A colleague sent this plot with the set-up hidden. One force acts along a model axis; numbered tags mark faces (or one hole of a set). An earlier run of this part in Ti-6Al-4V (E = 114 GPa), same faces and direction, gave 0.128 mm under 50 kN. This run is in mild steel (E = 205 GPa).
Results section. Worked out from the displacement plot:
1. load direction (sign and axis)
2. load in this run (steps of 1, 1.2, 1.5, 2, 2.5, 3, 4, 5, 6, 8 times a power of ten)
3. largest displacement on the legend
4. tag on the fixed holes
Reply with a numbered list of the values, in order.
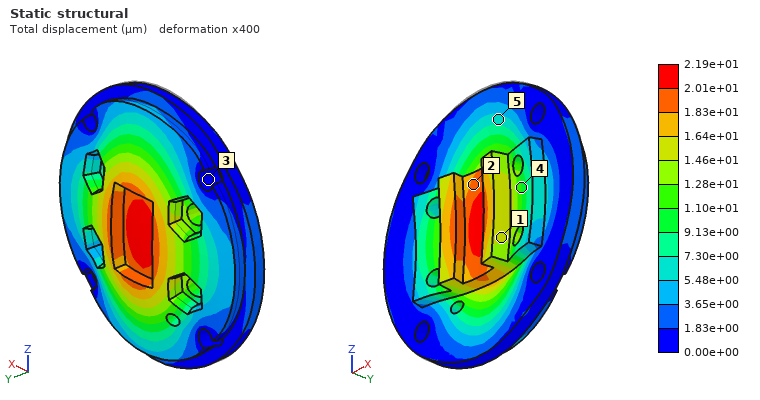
1. +Y
2. 15 kN
3. 2.19e+01 µm
4. 3
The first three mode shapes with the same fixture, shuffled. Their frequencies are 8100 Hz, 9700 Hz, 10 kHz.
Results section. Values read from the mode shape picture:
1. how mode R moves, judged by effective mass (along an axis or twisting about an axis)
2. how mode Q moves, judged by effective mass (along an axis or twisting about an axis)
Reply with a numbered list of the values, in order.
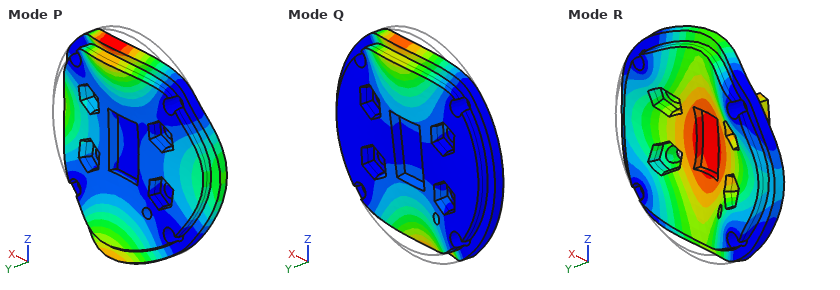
1. along Y
2. twisting about X
